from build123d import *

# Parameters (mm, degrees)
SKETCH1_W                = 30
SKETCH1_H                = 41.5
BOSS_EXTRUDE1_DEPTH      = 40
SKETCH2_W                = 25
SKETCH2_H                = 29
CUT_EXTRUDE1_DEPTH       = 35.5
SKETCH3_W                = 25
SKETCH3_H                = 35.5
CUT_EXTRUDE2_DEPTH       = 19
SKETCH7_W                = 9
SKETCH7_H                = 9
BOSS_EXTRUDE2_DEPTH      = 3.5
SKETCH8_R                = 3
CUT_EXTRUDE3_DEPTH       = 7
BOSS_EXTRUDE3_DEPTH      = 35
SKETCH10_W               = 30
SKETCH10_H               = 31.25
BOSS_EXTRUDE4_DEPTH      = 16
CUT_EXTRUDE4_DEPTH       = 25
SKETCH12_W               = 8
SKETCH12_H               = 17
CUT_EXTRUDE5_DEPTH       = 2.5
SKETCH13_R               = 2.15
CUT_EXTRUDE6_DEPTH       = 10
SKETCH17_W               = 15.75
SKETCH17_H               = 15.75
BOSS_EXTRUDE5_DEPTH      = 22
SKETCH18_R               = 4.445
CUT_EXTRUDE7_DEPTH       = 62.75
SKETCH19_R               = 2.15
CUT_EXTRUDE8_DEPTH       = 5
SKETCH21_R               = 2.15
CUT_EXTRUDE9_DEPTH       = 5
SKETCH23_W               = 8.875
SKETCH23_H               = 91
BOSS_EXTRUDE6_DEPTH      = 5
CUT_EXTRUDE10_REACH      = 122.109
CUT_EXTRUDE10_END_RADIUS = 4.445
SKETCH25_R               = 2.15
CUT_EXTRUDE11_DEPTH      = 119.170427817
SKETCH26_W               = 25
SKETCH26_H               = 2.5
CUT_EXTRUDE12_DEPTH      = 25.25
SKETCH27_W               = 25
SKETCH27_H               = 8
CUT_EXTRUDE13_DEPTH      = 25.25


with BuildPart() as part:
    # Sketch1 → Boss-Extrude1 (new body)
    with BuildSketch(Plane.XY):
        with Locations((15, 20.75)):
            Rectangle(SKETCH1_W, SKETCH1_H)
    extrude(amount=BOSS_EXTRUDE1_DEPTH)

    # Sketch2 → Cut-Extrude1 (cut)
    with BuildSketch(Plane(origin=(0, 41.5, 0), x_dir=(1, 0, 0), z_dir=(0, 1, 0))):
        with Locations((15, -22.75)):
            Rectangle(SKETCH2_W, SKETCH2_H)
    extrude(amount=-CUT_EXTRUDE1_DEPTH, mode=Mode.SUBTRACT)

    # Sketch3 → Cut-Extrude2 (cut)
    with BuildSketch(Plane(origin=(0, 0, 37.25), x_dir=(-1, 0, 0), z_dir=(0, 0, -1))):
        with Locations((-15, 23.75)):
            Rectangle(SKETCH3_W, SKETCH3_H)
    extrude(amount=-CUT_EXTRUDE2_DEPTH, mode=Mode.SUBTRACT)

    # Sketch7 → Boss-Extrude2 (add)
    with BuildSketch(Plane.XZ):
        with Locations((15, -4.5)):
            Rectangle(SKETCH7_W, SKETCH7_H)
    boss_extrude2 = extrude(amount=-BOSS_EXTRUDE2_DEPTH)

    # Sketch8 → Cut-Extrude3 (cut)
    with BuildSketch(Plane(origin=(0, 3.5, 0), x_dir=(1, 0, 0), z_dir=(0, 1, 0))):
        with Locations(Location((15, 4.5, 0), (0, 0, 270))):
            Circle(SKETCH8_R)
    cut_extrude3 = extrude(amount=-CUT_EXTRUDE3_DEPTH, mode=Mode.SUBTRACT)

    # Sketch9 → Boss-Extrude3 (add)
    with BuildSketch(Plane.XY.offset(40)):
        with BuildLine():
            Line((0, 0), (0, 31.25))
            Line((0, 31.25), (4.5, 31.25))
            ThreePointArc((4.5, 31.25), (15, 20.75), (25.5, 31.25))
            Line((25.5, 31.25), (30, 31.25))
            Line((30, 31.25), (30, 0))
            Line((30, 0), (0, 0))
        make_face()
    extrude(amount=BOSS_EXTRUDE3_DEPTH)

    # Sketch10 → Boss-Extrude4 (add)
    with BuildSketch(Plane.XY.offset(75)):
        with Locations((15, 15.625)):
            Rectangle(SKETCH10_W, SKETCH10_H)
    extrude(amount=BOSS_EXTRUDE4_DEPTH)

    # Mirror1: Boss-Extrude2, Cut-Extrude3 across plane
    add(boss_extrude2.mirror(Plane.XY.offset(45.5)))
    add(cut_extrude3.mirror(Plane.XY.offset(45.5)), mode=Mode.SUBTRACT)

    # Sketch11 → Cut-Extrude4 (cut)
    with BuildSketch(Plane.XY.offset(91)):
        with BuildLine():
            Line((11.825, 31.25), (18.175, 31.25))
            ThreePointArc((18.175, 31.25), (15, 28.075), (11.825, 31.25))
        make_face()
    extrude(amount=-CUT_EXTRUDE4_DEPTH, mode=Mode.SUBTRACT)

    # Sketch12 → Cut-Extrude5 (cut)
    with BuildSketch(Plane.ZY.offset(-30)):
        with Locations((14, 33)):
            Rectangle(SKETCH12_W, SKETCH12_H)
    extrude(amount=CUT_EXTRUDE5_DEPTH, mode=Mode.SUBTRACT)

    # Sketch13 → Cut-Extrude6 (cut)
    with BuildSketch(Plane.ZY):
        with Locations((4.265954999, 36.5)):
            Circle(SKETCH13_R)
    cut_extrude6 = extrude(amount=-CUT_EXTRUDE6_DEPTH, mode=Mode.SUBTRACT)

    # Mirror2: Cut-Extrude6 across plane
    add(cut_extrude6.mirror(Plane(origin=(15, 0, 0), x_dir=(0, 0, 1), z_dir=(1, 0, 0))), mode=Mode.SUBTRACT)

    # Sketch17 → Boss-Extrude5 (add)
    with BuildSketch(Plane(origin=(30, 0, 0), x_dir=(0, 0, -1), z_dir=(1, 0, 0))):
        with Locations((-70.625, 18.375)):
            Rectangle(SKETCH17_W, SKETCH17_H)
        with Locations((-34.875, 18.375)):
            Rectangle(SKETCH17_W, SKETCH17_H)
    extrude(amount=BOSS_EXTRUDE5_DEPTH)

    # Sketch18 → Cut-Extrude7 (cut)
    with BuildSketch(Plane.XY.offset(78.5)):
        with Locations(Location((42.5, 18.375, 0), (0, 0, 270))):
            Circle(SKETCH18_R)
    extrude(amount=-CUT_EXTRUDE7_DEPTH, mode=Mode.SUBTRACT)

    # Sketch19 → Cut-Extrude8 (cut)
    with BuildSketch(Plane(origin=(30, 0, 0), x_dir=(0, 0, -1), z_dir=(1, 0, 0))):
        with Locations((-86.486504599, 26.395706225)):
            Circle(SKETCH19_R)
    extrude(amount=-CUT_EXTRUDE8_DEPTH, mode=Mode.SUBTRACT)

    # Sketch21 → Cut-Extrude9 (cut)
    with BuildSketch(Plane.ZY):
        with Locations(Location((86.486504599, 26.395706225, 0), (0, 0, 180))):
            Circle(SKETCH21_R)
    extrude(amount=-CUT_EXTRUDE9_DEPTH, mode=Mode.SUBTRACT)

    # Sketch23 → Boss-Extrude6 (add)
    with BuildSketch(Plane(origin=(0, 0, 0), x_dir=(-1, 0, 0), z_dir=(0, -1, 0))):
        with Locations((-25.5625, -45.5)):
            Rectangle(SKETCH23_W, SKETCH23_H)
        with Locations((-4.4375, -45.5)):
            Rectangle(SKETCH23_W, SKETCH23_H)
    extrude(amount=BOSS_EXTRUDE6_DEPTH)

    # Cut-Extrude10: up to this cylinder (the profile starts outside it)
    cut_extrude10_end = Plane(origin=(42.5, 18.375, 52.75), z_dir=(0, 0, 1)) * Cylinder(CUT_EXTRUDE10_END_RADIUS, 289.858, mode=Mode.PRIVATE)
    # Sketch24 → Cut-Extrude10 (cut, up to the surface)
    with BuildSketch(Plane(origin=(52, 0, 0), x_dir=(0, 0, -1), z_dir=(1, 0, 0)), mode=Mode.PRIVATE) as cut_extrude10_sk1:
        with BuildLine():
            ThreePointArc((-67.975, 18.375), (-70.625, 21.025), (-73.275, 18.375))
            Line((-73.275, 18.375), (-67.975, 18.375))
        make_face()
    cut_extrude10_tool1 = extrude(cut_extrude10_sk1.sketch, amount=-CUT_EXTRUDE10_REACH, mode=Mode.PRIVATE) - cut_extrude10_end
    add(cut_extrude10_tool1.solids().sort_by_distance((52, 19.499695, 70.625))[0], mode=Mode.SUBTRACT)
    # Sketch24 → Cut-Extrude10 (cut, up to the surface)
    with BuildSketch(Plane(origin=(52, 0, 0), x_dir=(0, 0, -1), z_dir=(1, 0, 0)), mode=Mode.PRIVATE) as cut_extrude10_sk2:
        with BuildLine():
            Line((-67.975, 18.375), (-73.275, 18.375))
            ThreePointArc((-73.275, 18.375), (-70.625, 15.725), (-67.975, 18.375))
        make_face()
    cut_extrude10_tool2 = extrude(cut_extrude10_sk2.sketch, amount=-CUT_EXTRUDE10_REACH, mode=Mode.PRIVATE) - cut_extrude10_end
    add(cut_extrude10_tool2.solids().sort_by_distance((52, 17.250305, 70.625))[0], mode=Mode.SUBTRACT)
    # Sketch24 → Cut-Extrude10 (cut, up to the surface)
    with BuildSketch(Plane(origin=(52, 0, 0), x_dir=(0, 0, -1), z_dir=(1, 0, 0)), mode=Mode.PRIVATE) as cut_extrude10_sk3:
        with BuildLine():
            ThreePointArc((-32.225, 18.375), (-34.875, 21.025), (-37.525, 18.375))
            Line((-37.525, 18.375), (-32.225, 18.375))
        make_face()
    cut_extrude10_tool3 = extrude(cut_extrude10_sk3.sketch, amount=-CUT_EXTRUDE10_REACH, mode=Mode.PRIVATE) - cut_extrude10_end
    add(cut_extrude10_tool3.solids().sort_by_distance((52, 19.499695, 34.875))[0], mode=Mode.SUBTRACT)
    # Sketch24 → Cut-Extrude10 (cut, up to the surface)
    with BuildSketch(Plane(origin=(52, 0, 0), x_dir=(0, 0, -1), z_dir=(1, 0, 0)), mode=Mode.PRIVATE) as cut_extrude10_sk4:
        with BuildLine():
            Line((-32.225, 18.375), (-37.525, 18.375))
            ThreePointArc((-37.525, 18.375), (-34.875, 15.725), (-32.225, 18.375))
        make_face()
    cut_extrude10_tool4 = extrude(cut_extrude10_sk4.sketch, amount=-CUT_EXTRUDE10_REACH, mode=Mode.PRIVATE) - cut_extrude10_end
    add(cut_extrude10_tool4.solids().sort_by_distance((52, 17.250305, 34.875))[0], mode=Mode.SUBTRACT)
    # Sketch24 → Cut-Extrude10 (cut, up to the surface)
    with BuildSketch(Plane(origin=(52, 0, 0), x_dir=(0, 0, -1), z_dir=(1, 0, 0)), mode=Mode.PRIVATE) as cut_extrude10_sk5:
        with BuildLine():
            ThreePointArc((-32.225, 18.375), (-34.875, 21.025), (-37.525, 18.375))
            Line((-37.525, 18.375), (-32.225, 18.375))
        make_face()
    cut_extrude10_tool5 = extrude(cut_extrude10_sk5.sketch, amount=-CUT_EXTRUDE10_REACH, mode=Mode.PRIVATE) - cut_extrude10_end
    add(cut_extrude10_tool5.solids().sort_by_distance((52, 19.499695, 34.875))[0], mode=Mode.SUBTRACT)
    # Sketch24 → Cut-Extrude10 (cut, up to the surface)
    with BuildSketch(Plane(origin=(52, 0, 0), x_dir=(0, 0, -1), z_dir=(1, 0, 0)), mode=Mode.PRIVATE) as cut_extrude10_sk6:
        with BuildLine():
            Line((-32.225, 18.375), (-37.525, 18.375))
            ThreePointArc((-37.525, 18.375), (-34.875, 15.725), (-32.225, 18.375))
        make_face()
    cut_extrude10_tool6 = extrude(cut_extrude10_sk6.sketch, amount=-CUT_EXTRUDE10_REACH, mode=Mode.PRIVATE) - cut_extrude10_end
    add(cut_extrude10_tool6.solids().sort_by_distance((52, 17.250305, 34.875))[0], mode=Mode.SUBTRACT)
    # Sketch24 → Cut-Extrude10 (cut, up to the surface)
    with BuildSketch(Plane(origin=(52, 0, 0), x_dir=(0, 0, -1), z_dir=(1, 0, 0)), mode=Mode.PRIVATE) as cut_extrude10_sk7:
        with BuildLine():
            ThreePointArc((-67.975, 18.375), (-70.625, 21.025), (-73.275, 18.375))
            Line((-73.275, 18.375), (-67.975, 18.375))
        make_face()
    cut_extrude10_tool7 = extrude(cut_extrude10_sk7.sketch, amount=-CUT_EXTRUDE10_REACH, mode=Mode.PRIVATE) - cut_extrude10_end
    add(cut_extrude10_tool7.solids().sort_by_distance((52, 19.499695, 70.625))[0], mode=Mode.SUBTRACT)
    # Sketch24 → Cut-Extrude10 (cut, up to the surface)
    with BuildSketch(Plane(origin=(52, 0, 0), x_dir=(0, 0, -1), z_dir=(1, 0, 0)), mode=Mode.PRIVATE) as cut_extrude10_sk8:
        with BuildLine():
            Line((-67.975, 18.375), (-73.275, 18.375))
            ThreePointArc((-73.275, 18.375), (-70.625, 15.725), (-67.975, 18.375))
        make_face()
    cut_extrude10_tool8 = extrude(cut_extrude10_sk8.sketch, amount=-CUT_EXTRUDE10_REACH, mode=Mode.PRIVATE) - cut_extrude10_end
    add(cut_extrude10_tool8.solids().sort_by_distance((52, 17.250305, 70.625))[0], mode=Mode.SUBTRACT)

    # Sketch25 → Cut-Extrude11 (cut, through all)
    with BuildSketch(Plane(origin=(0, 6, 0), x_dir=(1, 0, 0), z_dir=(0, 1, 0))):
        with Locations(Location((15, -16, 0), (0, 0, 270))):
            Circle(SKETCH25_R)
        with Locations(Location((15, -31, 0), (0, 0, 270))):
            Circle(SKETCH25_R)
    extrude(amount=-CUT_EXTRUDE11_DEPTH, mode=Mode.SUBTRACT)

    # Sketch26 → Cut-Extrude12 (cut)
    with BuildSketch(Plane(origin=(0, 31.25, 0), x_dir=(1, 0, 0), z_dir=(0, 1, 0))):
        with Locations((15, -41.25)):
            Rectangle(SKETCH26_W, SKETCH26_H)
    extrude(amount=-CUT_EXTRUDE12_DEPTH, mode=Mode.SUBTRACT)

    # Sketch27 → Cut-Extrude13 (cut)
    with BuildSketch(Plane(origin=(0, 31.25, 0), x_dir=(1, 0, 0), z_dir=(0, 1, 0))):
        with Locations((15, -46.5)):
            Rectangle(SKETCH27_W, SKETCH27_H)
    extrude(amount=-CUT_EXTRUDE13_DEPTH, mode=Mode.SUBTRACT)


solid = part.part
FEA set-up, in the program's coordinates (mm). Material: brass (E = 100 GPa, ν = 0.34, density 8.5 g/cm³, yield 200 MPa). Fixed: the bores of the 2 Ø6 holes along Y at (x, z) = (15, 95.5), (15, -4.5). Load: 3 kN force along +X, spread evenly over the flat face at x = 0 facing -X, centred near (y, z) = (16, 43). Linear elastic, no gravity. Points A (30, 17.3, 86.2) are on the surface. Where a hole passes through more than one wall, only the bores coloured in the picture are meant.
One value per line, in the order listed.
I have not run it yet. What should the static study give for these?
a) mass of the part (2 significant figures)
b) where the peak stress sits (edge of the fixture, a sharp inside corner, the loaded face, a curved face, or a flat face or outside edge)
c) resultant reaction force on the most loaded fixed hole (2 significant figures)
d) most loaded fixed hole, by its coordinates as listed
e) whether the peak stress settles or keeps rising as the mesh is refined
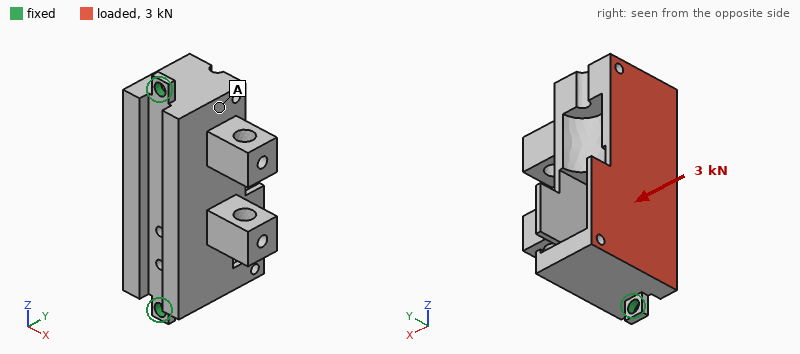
630 g
edge of the fixture
1.6 kN
(15, -4.5)
keeps rising
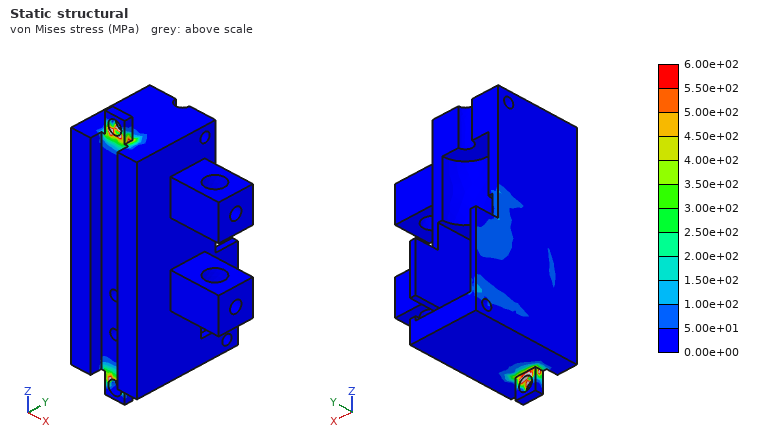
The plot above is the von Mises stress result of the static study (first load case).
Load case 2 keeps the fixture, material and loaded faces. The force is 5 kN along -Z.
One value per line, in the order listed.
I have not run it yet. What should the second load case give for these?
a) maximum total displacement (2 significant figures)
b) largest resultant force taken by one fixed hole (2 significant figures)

24 µm
2.9 kN
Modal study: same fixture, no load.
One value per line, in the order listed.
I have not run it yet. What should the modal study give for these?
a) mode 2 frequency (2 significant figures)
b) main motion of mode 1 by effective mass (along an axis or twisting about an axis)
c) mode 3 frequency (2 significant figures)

2300 Hz
along X
2400 Hz
